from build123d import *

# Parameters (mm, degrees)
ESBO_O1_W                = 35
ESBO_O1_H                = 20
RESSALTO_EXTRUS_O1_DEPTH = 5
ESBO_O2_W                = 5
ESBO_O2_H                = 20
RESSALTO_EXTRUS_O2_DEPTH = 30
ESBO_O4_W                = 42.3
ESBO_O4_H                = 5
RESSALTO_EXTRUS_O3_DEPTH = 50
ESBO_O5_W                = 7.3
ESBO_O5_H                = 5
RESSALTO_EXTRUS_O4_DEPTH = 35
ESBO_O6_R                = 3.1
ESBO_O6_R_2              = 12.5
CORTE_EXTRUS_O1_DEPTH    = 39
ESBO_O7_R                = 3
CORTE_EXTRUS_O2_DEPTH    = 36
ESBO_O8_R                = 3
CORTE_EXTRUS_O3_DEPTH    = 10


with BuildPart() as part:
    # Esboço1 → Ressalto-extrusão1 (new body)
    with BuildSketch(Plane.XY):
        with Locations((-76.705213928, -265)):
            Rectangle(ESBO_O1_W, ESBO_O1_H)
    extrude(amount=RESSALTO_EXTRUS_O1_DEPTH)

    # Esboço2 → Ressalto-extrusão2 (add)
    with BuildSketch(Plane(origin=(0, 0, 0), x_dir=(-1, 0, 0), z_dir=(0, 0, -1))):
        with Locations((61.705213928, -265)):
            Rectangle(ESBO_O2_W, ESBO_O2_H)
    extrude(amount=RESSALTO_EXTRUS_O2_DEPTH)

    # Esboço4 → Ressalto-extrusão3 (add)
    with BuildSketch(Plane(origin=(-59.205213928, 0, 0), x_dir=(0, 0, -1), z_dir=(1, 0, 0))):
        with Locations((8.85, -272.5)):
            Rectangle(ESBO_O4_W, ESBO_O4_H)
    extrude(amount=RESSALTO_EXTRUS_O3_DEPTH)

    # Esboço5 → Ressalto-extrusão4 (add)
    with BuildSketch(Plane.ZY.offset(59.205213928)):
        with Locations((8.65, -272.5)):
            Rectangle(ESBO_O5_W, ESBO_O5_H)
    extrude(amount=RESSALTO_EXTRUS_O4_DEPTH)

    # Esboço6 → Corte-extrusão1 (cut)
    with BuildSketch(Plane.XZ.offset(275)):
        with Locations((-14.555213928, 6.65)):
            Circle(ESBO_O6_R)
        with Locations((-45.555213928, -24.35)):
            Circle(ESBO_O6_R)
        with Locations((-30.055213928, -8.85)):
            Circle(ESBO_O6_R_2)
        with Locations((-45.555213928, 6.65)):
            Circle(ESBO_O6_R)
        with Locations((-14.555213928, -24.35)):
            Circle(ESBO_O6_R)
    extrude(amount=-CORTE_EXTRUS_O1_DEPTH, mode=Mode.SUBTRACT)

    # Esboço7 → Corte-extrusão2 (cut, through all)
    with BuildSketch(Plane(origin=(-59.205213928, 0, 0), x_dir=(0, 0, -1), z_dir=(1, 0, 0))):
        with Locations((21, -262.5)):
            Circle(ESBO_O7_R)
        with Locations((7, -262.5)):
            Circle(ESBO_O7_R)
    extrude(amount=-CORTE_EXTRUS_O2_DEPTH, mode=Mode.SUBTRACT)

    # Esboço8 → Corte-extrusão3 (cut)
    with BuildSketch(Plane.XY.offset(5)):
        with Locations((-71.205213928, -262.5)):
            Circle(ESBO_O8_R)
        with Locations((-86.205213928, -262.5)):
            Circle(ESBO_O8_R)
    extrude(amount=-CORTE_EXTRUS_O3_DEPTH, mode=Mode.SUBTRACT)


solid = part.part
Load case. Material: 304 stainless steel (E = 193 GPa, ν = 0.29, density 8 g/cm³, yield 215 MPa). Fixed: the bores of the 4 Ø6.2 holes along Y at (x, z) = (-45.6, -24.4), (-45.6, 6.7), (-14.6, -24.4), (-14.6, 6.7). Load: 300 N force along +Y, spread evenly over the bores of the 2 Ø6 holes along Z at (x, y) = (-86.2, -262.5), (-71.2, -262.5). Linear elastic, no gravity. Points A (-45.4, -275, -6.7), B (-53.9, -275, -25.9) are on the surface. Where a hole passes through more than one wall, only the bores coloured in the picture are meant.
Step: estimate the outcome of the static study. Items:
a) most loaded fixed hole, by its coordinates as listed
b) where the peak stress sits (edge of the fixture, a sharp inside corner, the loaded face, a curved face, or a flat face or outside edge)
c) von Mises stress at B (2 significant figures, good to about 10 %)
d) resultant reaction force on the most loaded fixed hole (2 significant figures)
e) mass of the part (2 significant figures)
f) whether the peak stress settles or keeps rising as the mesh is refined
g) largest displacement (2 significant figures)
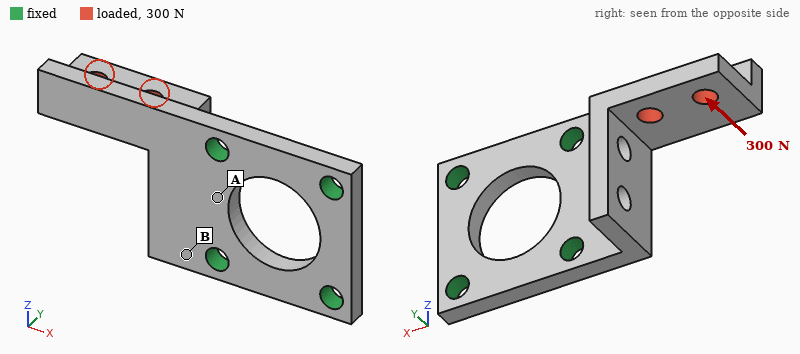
(-45.6, 6.7)
edge of the fixture
35 MPa
270 N
120 g
keeps rising
86 µm
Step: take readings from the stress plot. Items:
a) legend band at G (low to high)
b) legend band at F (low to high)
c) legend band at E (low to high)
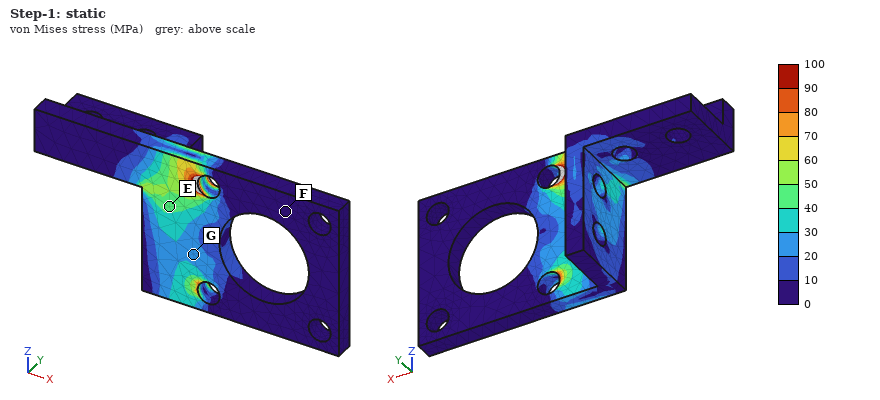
20 to 30 MPa
0 to 10 MPa
40 to 50 MPa
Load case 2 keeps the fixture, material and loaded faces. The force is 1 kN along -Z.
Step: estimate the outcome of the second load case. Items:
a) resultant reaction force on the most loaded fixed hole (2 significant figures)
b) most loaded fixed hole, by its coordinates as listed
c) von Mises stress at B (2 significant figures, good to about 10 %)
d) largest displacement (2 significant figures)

1.3 kN
(-45.6, -24.4)
15 MPa
76 µm
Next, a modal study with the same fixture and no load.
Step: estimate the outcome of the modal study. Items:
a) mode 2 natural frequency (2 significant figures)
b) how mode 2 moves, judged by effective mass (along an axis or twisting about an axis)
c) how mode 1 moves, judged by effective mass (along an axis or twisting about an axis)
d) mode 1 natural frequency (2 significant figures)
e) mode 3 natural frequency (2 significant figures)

4900 Hz
along Z
along Y
1900 Hz
7300 Hz
